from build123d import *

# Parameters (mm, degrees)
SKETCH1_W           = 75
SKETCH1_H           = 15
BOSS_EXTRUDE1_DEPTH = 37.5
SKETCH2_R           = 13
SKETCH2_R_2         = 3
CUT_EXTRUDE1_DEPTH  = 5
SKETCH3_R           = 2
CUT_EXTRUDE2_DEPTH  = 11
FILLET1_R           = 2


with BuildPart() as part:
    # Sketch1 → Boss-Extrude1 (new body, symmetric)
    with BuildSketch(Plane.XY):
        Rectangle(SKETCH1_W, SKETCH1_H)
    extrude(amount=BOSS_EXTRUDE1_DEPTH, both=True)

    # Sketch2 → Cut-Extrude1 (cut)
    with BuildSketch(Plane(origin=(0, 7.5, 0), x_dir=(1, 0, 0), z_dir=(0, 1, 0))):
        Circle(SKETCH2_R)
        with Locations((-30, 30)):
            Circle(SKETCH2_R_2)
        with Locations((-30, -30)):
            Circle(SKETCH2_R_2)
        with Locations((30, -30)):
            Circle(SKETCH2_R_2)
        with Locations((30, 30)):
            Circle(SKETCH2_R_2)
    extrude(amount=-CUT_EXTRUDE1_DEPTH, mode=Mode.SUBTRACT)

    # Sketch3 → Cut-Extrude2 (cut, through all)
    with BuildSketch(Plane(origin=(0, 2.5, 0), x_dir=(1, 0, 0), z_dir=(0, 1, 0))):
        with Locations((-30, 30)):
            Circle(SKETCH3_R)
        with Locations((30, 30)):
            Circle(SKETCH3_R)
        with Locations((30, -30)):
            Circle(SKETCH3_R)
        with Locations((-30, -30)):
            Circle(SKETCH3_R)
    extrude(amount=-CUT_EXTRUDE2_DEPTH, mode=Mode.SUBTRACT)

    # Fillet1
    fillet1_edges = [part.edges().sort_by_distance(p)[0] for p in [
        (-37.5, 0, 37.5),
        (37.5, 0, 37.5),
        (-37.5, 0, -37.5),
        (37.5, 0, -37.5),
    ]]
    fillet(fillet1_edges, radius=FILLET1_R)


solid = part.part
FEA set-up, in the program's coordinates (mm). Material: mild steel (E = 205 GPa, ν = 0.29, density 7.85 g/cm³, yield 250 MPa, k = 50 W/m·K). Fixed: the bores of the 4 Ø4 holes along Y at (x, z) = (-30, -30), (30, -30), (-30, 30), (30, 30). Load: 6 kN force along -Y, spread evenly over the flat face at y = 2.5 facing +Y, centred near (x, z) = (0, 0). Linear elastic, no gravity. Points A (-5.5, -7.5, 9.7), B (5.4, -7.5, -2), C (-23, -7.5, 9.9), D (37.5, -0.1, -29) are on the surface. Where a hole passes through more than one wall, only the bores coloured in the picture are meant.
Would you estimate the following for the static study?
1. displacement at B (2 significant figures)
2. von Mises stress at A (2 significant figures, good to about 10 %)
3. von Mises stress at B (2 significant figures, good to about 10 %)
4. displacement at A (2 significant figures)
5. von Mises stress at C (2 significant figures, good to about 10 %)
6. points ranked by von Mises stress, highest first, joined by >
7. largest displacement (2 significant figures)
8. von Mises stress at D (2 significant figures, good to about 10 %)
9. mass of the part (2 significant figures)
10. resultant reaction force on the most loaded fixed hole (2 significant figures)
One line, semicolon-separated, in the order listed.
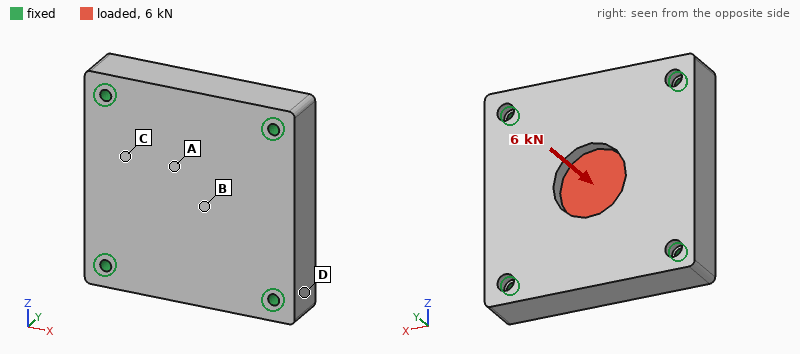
10 µm; 26 MPa; 35 MPa; 8.9 µm; 12 MPa; B > A > C > D; 11 µm; 7.4 MPa; 630 g; 1.6 kN
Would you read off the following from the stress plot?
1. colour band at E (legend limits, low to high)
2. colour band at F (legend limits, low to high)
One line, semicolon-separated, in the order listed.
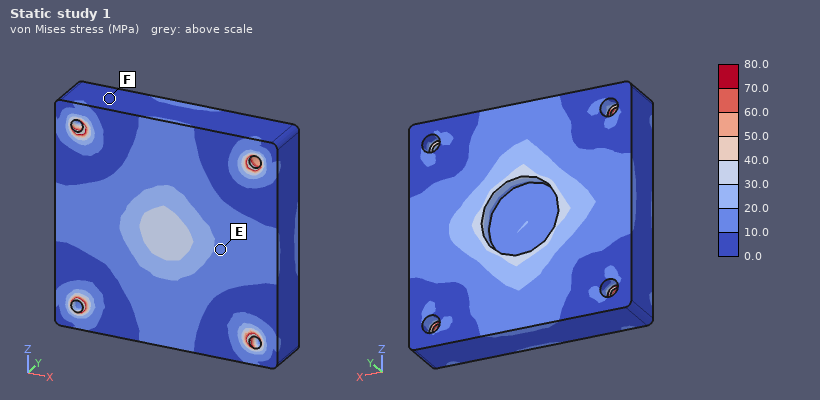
10.0 to 20.0 MPa; 0.0 to 10.0 MPa
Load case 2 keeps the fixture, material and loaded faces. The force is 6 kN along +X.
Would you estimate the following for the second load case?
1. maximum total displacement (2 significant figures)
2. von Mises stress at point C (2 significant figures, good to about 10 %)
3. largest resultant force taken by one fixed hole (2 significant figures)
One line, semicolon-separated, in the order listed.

2.4 µm; 5.4 MPa; 1.7 kN
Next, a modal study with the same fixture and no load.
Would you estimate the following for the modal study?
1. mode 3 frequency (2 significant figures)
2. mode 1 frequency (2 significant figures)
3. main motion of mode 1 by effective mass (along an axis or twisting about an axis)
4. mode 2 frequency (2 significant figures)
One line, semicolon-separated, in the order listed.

15 kHz; 9100 Hz; along Y; 15 kHz
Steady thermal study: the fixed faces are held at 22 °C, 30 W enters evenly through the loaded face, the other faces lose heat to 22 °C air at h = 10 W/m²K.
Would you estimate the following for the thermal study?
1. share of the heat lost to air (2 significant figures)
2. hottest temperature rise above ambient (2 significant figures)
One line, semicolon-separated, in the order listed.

3.4 %; 21 K
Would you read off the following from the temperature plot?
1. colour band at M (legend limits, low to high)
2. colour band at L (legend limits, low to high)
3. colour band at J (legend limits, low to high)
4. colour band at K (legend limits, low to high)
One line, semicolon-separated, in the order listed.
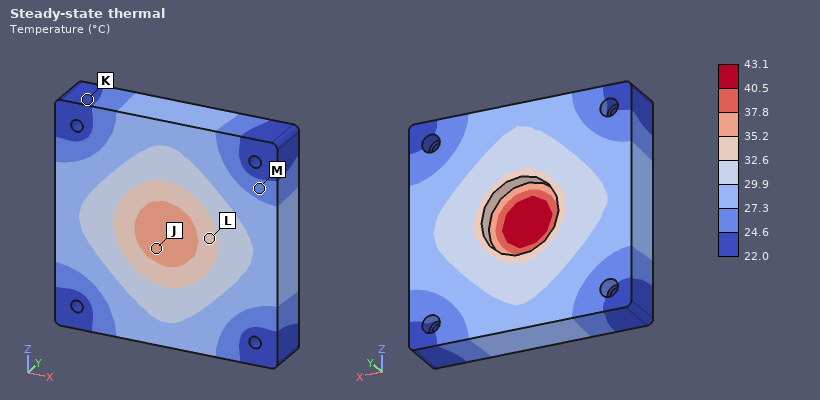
24.6 to 27.3 °C; 32.6 to 35.2 °C; 35.2 to 37.8 °C; 22.0 to 24.6 °C
